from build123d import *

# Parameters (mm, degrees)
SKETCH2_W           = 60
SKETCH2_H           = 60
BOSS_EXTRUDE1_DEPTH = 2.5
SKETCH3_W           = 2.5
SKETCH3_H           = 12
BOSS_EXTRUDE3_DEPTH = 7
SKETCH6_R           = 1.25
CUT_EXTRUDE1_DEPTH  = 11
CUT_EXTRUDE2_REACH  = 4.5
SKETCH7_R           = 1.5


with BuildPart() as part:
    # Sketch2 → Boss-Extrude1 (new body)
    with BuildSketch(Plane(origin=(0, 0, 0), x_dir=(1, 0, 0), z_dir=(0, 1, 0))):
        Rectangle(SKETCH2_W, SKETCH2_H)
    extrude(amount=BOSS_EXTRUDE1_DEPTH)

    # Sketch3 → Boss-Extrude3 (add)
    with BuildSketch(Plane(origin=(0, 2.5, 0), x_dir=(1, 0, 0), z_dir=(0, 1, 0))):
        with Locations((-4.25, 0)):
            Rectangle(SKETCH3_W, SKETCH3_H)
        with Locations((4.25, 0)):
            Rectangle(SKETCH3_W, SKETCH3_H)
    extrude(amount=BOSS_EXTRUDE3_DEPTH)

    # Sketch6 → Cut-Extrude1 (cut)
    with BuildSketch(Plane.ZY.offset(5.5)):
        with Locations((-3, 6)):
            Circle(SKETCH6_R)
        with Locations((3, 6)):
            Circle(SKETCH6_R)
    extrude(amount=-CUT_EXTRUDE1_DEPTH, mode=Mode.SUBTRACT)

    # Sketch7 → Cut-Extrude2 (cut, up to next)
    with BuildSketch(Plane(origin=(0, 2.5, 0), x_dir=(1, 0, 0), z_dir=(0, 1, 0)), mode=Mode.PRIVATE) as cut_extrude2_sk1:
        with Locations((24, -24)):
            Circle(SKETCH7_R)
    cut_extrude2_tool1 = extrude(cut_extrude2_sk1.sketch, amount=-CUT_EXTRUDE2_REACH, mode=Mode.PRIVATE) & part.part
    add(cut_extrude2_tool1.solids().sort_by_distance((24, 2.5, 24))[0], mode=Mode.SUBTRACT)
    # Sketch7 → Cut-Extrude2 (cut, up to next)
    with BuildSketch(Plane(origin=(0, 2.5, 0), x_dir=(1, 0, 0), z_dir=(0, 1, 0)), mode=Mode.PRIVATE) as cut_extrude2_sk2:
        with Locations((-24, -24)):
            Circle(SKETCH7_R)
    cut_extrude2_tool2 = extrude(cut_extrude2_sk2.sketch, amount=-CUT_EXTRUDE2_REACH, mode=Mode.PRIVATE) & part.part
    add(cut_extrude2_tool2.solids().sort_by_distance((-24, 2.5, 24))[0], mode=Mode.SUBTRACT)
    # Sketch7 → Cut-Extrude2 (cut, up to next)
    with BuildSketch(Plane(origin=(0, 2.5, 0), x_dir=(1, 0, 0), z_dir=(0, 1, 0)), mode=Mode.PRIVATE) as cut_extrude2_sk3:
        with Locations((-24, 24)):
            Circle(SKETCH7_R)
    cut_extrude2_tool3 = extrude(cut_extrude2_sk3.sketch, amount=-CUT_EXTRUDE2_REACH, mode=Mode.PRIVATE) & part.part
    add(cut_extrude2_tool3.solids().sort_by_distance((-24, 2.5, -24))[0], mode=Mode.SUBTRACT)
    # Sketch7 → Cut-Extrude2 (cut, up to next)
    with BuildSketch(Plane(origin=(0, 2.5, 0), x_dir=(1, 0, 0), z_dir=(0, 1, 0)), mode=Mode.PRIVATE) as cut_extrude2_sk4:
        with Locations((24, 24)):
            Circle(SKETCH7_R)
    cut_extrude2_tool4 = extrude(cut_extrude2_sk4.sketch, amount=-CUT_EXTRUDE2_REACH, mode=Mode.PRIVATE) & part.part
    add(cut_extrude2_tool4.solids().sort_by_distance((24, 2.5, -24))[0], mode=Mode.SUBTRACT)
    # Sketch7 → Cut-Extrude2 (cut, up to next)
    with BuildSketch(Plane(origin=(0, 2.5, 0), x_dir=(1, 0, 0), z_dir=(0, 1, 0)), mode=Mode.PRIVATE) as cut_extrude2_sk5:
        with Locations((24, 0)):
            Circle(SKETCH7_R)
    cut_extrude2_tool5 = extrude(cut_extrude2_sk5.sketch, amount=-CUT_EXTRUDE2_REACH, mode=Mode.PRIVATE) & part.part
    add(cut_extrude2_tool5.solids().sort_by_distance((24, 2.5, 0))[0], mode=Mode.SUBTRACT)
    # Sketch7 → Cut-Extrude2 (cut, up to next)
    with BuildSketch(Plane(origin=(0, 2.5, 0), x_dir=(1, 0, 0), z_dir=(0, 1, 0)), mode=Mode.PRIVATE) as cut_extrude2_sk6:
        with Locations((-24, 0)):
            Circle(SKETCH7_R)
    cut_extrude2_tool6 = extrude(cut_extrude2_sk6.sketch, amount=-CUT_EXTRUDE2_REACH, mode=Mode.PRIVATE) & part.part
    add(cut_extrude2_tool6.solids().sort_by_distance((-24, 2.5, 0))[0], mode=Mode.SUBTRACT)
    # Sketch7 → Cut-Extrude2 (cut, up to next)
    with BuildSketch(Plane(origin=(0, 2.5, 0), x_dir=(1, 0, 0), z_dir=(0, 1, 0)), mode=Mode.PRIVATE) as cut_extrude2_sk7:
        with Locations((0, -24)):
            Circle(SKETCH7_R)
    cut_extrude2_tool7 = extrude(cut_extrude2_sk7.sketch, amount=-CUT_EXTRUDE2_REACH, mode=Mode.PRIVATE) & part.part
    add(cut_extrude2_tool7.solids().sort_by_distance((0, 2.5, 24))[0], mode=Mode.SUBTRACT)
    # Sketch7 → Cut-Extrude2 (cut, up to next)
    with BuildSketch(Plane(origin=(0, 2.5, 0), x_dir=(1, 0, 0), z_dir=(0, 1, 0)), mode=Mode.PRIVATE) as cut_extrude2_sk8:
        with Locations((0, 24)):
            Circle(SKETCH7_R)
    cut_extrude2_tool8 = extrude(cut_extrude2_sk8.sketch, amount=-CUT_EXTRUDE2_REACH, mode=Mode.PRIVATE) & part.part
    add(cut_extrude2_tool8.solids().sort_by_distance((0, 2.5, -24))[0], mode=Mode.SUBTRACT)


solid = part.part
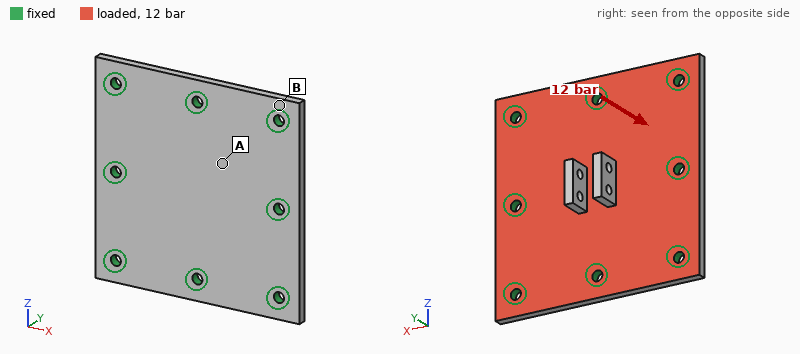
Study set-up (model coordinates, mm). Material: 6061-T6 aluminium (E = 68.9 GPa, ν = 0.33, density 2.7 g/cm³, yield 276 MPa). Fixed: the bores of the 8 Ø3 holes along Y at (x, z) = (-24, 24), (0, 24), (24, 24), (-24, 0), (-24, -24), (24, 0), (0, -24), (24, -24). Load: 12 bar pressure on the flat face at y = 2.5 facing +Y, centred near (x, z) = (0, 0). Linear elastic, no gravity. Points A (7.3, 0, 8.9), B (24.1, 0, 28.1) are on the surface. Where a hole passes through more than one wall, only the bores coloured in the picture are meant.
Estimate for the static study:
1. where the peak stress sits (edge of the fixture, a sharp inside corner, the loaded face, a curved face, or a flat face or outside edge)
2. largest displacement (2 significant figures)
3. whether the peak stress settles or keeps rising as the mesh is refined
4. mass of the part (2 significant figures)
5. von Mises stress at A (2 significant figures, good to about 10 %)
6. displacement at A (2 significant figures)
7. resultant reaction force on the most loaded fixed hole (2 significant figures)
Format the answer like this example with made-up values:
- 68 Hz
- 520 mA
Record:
- edge of the fixture
- 82 µm
- keeps rising
- 25 g
- 51 MPa
- 64 µm
- 700 N
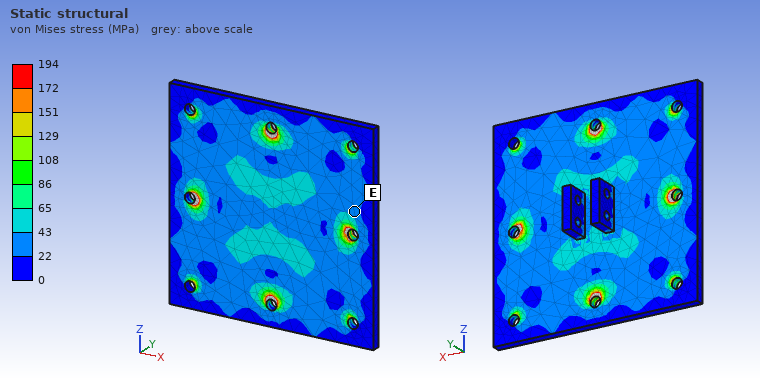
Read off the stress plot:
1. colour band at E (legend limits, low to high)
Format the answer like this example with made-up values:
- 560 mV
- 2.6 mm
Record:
- 22 to 43 MPa
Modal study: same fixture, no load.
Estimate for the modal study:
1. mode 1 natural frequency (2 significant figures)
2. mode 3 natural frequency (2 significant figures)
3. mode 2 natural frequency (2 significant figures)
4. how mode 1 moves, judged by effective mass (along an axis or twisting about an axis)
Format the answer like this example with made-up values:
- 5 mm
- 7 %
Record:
- 7800 Hz
- 14 kHz
- 14 kHz
- along Y
